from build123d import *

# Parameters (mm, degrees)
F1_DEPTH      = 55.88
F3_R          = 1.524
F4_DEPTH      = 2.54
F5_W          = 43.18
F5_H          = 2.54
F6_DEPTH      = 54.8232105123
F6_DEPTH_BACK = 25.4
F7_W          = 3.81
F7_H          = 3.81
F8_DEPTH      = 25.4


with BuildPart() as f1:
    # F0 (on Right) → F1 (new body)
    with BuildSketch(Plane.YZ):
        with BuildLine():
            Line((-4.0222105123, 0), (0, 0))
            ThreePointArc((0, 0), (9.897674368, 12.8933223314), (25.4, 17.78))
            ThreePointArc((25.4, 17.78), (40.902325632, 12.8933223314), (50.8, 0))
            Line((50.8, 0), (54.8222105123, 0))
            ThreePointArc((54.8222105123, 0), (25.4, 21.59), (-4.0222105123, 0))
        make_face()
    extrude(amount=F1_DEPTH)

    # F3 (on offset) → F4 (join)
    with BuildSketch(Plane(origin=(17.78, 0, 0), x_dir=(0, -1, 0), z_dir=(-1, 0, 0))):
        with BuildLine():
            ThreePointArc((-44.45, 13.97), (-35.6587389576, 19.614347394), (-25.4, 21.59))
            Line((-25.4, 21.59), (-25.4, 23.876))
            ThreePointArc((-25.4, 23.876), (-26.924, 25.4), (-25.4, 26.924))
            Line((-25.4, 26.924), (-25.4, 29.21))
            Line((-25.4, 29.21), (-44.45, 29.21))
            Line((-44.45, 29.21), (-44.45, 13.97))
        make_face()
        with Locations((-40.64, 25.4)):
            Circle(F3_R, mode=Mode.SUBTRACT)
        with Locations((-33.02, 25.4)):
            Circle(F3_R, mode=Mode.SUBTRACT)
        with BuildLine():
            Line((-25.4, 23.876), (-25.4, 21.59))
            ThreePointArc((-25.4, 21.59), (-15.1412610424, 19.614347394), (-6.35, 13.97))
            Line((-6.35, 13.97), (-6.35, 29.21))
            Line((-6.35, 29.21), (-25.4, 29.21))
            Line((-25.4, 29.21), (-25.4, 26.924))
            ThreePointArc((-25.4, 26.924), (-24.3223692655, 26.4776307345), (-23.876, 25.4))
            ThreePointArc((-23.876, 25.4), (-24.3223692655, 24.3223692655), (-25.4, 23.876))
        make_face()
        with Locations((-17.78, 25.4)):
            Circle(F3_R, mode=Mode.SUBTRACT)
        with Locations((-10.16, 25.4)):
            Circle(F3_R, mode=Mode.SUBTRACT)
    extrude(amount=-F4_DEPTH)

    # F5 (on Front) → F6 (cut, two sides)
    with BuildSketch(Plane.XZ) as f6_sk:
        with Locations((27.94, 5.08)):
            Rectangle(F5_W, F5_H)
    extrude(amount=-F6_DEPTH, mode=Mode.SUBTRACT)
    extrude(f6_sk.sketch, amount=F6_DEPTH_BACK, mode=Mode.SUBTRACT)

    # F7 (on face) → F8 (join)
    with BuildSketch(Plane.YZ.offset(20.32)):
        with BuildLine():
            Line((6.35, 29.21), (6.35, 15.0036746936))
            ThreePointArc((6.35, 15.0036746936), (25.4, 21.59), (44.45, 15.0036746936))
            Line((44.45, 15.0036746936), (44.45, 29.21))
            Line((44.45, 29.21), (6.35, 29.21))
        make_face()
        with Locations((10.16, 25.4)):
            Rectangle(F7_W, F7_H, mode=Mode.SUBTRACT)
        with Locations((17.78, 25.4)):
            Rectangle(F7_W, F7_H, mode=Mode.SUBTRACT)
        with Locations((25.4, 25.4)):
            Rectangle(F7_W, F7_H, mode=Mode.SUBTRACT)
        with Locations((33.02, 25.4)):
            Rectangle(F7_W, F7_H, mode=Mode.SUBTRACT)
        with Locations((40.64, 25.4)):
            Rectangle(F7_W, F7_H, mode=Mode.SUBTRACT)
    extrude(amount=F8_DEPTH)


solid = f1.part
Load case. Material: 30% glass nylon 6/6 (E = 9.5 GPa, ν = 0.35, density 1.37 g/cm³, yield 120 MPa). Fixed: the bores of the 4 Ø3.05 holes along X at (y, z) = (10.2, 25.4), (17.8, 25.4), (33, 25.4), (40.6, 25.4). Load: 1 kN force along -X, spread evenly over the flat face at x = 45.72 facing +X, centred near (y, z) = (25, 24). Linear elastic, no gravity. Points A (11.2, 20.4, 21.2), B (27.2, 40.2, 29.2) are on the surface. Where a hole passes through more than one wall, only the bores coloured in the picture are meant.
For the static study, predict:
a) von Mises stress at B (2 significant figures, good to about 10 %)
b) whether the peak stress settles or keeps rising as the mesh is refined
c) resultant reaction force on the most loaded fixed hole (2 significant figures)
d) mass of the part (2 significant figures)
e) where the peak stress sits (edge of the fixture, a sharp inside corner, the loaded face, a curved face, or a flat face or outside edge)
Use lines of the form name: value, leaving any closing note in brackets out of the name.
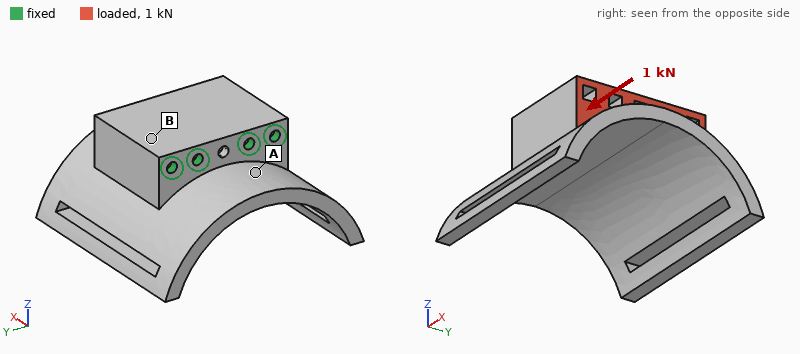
von Mises stress at B: 3.8 MPa
whether the peak stress settles or keeps rising as the mesh is refined: keeps rising
resultant reaction force on the most loaded fixed hole: 260 N
mass of the part: 31 g
where the peak stress sits: edge of the fixture
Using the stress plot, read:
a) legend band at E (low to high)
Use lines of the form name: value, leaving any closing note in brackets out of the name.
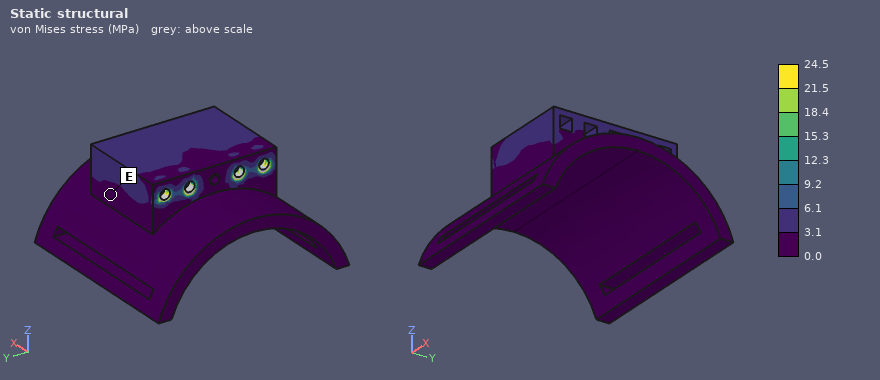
legend band at E: 0.0 to 3.1 MPa
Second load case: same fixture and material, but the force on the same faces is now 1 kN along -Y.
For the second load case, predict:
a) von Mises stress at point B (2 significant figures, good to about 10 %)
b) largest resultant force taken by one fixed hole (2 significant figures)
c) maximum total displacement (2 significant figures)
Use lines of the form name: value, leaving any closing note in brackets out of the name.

von Mises stress at point B: 12 MPa
largest resultant force taken by one fixed hole: 740 N
maximum total displacement: 0.10 mm
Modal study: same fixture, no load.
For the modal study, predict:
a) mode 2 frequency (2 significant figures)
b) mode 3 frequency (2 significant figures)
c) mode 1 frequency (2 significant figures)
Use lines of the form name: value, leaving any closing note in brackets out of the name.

mode 2 frequency: 2300 Hz
mode 3 frequency: 2300 Hz
mode 1 frequency: 1200 Hz
